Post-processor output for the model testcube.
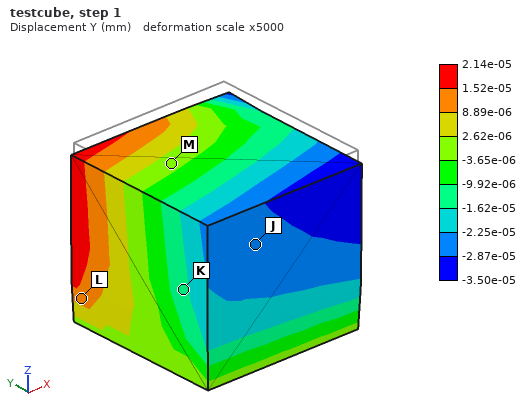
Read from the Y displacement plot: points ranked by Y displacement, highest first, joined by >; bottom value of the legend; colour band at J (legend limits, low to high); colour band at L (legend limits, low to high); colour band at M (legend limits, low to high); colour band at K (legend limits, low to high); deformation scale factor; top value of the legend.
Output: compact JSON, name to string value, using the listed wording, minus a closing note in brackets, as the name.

{"points ranked by Y displacement, highest first, joined by >": "L > M > K > J", "bottom value of the legend": "-3.50e-05 mm", "colour band at J": "-2.87e-05 to -2.25e-05 mm", "colour band at L": "8.89e-06 to 1.52e-05 mm", "colour band at M": "-3.65e-06 to 2.62e-06 mm", "colour band at K": "-1.62e-05 to -9.92e-06 mm", "deformation scale factor": "5000", "top value of the legend": "2.14e-05 mm"}
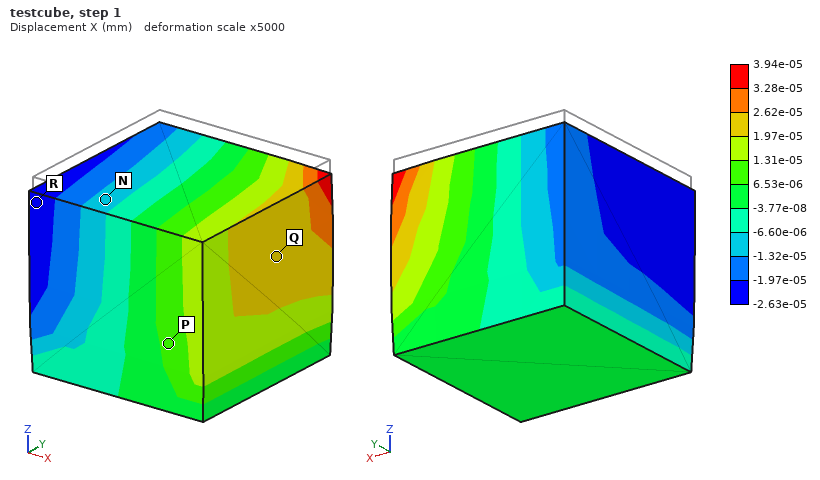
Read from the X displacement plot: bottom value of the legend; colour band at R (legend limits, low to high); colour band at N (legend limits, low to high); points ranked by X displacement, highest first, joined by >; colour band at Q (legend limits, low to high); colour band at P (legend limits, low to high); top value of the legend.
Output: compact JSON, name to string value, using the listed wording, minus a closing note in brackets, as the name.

{"bottom value of the legend": "-2.63e-05 mm", "colour band at R": "-2.63e-05 to -1.97e-05 mm", "colour band at N": "-1.32e-05 to -6.60e-06 mm", "points ranked by X displacement, highest first, joined by >": "Q > P > N > R", "colour band at Q": "1.97e-05 to 2.62e-05 mm", "colour band at P": "6.53e-06 to 1.31e-05 mm", "top value of the legend": "3.94e-05 mm"}
